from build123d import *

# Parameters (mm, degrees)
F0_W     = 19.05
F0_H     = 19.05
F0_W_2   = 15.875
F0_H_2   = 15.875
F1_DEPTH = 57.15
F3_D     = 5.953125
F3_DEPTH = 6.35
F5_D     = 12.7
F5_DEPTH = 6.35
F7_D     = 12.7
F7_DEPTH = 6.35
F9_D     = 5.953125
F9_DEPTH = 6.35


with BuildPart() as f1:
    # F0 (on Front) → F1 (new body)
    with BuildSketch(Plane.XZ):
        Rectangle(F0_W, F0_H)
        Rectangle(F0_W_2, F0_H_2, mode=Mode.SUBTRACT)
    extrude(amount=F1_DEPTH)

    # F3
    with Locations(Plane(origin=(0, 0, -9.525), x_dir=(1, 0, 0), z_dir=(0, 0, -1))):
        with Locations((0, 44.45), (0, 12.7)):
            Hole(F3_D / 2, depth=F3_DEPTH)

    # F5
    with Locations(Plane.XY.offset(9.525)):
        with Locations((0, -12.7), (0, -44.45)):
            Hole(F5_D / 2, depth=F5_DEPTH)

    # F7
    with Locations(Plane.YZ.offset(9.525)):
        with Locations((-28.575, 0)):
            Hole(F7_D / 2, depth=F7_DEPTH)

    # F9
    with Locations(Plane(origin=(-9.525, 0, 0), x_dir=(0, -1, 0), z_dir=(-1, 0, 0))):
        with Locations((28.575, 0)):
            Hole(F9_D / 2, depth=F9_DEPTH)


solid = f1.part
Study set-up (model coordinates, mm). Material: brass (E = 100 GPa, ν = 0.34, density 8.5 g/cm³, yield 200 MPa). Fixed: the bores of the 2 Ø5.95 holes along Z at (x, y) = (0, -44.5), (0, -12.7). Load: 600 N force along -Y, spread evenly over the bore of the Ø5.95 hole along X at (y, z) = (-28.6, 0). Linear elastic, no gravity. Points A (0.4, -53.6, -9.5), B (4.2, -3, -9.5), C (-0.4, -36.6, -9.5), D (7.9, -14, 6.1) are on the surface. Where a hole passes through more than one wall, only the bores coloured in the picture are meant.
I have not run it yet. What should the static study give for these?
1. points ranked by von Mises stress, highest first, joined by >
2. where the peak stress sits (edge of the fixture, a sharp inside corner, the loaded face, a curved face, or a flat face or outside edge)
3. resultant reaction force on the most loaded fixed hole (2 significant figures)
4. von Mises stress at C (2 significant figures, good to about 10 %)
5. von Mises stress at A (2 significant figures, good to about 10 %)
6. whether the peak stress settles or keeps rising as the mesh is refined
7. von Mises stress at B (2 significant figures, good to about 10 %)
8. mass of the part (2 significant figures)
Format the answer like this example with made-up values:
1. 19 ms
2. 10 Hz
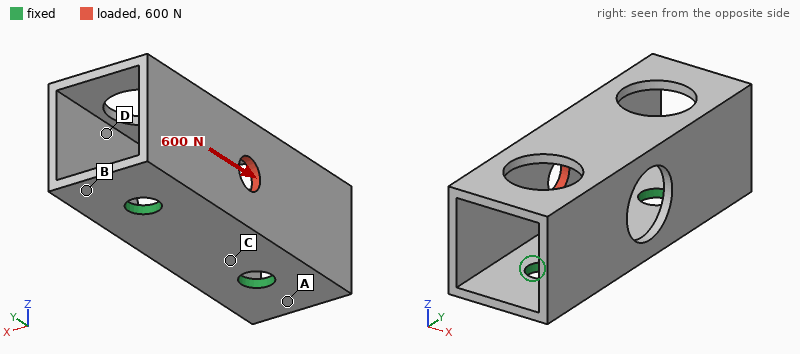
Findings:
1. A > B > C > D
2. edge of the fixture
3. 360 N
4. 8.9 MPa
5. 22 MPa
6. keeps rising
7. 17 MPa
8. 48 g
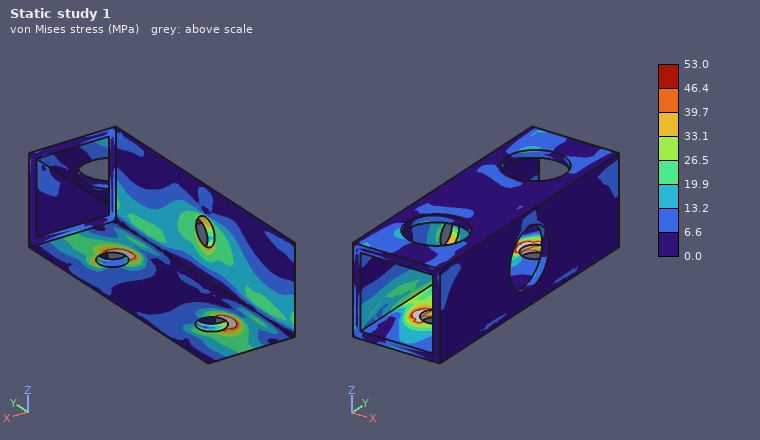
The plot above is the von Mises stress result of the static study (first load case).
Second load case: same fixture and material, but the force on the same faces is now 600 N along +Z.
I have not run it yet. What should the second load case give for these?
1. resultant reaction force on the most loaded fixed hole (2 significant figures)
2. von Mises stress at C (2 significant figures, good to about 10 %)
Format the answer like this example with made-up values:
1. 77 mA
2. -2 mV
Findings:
1. 320 N
2. 40 MPa
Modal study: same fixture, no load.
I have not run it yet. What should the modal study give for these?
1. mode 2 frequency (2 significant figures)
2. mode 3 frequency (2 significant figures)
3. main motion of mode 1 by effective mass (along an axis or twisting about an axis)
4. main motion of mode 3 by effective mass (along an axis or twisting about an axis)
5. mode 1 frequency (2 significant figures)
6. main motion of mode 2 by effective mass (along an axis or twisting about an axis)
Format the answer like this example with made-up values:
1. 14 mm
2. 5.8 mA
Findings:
1. 4000 Hz
2. 4500 Hz
3. along X
4. twisting about Z
5. 1600 Hz
6. along Y
